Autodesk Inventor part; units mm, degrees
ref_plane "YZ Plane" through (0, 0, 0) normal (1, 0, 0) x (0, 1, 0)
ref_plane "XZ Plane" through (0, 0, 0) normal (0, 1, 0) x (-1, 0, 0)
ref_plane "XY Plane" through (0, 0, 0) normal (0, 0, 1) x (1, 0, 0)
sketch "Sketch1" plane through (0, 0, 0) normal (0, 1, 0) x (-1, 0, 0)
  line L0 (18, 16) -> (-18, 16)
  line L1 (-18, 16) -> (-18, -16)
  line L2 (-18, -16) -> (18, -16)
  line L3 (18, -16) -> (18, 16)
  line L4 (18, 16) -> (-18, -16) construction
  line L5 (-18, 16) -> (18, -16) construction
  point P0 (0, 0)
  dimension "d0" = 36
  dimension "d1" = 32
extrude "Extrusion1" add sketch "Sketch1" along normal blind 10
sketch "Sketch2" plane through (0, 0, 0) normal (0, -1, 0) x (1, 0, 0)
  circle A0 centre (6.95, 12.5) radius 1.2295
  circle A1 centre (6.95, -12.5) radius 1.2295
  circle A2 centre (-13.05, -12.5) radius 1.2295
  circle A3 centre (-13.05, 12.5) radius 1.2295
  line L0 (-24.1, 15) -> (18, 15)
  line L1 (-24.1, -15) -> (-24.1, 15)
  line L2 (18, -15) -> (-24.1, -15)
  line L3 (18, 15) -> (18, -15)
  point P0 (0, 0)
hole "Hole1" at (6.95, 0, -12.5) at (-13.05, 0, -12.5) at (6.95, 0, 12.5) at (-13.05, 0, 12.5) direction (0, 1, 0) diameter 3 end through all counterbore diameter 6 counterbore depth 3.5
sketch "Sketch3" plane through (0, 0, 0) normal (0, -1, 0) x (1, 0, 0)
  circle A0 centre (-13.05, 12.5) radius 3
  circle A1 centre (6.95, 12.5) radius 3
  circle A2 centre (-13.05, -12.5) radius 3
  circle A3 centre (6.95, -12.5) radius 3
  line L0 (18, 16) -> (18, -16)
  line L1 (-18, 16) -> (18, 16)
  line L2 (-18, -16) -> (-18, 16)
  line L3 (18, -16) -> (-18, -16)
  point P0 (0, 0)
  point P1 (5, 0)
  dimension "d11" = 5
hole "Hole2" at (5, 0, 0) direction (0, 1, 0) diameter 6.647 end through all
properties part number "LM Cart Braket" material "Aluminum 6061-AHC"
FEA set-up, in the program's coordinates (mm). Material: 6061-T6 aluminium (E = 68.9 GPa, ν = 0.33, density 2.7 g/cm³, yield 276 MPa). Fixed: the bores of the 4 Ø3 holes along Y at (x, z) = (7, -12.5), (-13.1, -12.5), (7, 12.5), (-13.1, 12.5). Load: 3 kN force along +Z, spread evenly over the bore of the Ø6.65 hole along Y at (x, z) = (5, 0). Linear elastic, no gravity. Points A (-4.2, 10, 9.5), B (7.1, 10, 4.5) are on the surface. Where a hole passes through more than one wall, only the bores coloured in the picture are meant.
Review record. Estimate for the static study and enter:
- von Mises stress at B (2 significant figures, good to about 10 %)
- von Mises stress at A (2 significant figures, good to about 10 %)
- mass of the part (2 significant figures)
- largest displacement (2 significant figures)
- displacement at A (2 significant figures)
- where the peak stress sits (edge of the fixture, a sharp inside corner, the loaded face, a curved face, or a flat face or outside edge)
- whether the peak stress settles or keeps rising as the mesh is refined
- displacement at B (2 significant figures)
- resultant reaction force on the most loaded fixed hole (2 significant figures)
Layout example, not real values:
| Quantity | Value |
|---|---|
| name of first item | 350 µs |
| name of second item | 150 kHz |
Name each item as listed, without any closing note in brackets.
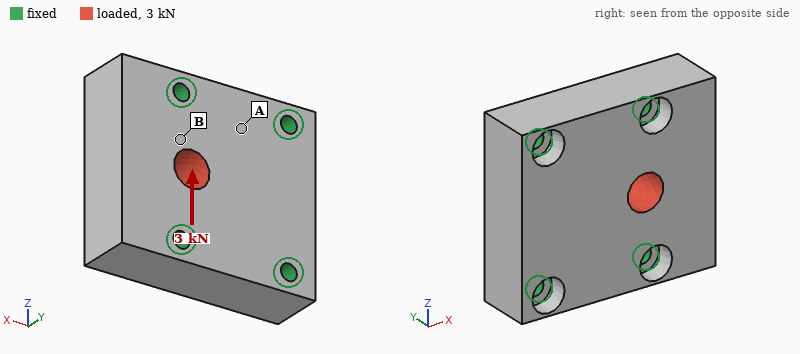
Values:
| Quantity | Value |
|---|---|
| von Mises stress at B | 17 MPa |
| von Mises stress at A | 5.0 MPa |
| mass of the part | 29 g |
| largest displacement | 2.9 µm |
| displacement at A | 1.1 µm |
| where the peak stress sits | edge of the fixture |
| whether the peak stress settles or keeps rising as the mesh is refined | keeps rising |
| displacement at B | 1.9 µm |
| resultant reaction force on the most loaded fixed hole | 1.2 kN |
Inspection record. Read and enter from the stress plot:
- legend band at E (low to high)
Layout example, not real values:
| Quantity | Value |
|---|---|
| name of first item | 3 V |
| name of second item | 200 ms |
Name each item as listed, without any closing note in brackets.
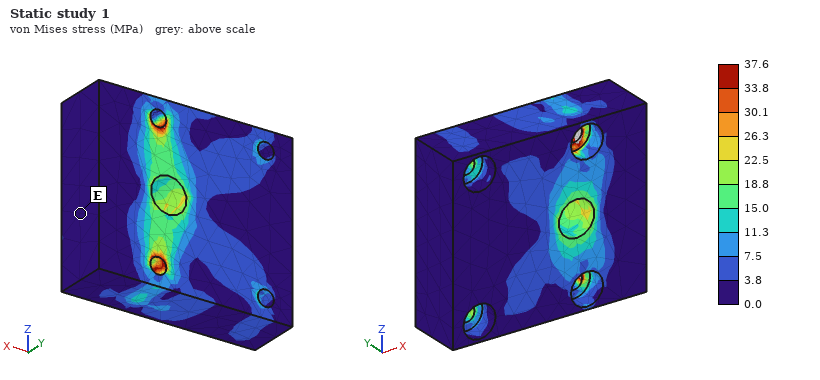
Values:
| Quantity | Value |
|---|---|
| legend band at E | 0.0 to 3.8 MPa |
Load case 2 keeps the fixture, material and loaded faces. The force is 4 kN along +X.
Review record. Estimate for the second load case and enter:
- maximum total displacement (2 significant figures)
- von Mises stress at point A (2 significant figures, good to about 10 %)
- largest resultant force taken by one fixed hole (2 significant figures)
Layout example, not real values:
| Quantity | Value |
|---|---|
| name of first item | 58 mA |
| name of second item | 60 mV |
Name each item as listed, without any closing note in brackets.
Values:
| Quantity | Value |
|---|---|
| maximum total displacement | 6.1 µm |
| von Mises stress at point A | 11 MPa |
| largest resultant force taken by one fixed hole | 1.2 kN |
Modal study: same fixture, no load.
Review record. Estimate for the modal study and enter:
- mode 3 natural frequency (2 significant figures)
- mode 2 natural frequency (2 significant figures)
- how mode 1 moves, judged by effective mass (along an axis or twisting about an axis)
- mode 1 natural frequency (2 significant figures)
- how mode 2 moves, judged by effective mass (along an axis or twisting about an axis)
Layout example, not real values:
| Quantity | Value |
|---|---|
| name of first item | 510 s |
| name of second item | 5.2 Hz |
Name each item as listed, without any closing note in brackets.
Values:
| Quantity | Value |
|---|---|
| mode 3 natural frequency | 42 kHz |
| mode 2 natural frequency | 36 kHz |
| how mode 1 moves, judged by effective mass | along Y |
| mode 1 natural frequency | 26 kHz |
| how mode 2 moves, judged by effective mass | along Y |
